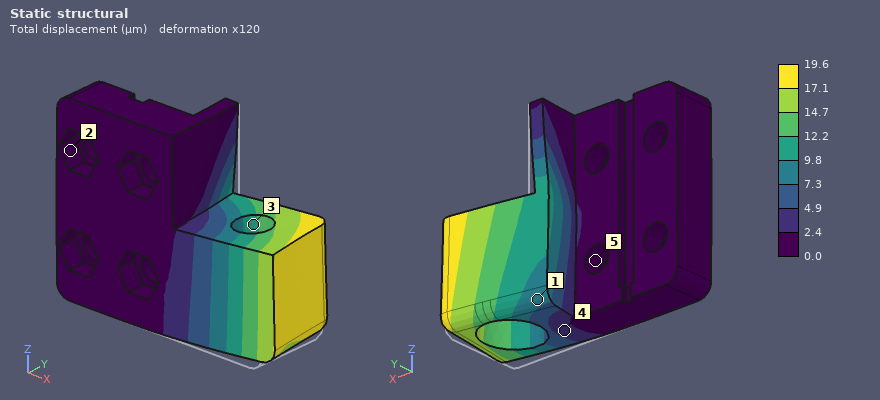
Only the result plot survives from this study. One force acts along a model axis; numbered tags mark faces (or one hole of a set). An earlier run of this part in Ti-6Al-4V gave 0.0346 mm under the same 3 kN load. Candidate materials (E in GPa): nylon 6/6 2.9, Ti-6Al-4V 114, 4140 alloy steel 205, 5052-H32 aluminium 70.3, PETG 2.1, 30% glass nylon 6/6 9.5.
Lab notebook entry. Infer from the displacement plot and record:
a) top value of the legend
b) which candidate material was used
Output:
19.6 µm
4140 alloy steel
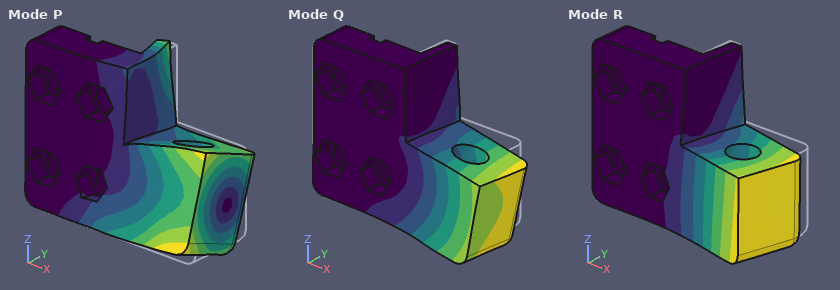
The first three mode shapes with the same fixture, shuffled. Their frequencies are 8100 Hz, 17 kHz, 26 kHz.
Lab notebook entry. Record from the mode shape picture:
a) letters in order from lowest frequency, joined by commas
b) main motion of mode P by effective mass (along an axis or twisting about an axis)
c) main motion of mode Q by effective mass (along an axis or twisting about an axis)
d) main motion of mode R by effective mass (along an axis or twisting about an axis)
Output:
R, Q, P
twisting about X
along Z
along Y
